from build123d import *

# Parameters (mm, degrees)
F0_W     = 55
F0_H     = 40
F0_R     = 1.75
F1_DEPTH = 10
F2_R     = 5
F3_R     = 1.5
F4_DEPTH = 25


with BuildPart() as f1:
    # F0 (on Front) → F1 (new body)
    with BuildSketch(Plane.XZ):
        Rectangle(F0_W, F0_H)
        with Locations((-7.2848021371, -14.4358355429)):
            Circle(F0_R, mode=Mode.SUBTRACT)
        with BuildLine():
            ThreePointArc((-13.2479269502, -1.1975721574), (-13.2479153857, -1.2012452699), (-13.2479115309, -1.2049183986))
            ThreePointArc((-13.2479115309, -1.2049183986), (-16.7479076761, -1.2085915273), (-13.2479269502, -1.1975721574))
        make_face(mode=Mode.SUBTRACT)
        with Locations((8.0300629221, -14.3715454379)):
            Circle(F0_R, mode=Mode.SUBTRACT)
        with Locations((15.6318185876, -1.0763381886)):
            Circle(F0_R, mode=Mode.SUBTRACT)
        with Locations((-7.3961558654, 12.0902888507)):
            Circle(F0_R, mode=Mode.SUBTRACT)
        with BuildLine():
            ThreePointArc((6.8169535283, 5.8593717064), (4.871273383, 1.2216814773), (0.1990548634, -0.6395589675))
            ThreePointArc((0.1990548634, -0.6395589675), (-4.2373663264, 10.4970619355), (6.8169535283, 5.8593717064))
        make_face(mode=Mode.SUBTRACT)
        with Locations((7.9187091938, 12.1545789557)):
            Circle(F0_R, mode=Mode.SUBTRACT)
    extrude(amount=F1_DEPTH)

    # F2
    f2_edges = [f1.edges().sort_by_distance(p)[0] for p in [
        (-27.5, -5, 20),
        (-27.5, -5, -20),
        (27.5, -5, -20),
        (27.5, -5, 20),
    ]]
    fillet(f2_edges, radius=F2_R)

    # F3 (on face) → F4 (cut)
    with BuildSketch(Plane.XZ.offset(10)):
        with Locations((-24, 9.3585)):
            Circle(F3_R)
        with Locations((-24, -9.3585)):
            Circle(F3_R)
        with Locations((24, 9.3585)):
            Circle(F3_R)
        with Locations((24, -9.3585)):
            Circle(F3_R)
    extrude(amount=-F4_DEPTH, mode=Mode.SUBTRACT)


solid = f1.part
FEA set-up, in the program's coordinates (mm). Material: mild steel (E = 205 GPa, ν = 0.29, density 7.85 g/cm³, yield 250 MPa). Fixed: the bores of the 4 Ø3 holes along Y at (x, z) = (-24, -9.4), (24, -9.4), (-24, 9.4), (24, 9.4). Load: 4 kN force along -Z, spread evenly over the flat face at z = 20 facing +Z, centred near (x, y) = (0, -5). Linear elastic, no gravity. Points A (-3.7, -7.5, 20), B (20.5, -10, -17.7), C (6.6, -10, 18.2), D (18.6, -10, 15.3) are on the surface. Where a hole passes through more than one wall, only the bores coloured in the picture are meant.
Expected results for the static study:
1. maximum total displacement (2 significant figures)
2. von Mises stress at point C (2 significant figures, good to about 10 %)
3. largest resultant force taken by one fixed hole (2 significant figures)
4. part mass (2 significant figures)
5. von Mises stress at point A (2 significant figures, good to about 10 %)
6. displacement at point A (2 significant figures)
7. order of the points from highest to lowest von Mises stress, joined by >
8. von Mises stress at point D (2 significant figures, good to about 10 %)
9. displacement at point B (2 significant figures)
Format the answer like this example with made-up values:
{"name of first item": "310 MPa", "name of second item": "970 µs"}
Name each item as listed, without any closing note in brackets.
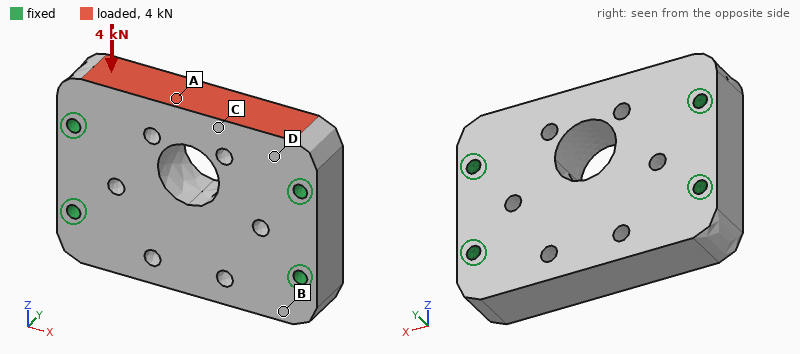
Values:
{"maximum total displacement": "2.9 µm", "von Mises stress at point C": "13 MPa", "largest resultant force taken by one fixed hole": "1.2 kN", "part mass": "150 g", "von Mises stress at point A": "17 MPa", "displacement at point A": "2.8 µm", "order of the points from highest to lowest von Mises stress, joined by >": "A > C > D > B", "von Mises stress at point D": "9.0 MPa", "displacement at point B": "0.45 µm"}
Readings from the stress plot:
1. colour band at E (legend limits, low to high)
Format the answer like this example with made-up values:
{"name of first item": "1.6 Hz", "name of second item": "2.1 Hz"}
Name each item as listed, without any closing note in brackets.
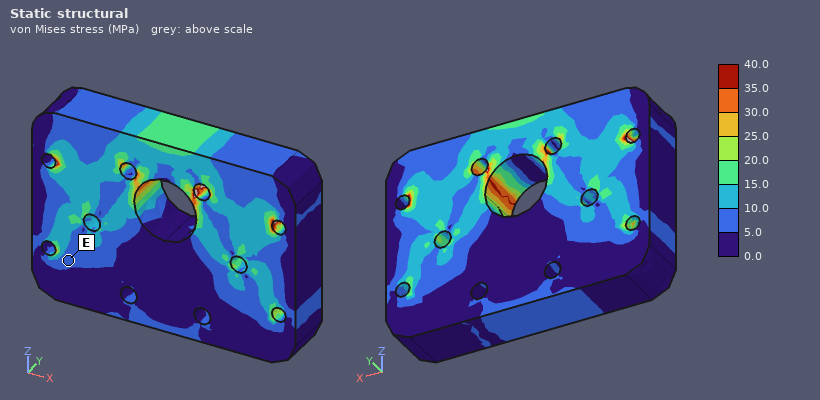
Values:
{"colour band at E": "5.0 to 10.0 MPa"}
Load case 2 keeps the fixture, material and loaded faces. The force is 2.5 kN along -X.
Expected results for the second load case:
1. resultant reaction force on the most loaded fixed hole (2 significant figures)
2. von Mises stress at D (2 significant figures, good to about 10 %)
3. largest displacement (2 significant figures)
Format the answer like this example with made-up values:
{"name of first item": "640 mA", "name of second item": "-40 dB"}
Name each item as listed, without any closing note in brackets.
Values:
{"resultant reaction force on the most loaded fixed hole": "1.3 kN", "von Mises stress at D": "12 MPa", "largest displacement": "1.3 µm"}
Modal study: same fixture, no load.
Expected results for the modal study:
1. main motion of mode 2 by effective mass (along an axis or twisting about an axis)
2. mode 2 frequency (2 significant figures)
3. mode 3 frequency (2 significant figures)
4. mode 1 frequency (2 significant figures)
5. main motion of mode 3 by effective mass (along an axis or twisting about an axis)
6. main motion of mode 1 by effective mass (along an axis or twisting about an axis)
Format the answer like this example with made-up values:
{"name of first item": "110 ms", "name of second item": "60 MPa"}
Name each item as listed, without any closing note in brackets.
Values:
{"main motion of mode 2 by effective mass": "twisting about X", "mode 2 frequency": "18 kHz", "mode 3 frequency": "26 kHz", "mode 1 frequency": "16 kHz", "main motion of mode 3 by effective mass": "along Z", "main motion of mode 1 by effective mass": "along Y"}
